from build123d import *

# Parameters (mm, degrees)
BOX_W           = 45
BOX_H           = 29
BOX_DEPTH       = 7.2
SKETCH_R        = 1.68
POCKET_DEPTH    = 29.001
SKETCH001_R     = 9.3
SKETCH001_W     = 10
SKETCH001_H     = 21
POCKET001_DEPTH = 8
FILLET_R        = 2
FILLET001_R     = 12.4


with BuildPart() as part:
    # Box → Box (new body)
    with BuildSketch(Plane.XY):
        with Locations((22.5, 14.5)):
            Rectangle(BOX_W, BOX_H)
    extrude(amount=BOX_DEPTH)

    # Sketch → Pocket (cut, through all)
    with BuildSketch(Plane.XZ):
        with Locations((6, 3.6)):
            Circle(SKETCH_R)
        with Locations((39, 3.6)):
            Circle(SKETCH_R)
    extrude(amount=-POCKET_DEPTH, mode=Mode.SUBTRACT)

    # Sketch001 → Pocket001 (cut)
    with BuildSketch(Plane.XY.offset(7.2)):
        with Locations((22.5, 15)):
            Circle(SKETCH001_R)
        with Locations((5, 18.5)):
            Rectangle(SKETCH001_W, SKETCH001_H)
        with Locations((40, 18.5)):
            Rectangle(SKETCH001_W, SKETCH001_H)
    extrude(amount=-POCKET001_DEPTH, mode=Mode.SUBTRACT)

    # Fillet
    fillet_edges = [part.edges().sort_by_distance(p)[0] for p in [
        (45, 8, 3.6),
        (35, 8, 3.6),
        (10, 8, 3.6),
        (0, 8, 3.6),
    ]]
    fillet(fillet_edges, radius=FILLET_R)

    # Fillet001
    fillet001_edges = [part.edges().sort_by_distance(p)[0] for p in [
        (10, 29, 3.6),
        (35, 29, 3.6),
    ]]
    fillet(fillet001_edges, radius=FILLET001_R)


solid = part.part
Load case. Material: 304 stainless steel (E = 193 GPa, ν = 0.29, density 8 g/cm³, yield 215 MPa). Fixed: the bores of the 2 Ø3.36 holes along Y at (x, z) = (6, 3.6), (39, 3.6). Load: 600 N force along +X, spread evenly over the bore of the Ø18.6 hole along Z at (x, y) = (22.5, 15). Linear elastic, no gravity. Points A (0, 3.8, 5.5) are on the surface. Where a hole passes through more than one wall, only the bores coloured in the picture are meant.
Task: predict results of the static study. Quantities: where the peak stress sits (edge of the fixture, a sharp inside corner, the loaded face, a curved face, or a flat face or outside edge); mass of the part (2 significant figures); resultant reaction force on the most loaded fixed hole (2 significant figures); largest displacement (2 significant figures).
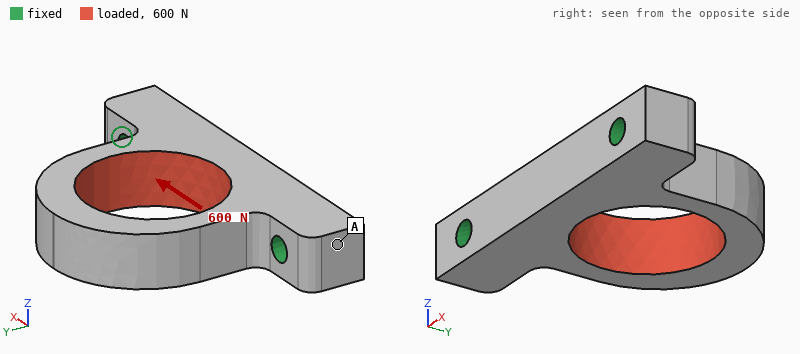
a curved face
30 g
350 N
8.1 µm
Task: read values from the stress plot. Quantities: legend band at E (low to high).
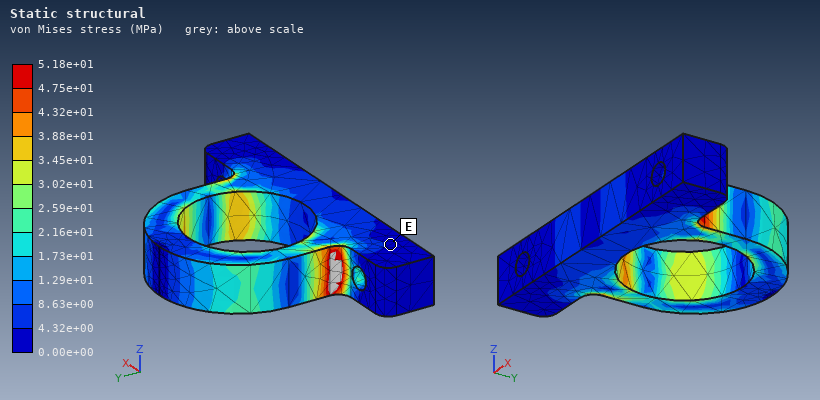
0.00e+00 to 4.32e+00 MPa
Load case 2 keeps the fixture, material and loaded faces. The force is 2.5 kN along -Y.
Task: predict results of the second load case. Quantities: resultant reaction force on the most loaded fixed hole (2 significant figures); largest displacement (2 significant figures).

1.3 kN
6.1 µm
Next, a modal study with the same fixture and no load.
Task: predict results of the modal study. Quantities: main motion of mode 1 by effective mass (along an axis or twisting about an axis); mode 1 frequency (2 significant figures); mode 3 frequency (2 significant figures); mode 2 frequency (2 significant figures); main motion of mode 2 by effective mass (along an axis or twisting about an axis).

along Z
6600 Hz
17 kHz
11 kHz
along X
